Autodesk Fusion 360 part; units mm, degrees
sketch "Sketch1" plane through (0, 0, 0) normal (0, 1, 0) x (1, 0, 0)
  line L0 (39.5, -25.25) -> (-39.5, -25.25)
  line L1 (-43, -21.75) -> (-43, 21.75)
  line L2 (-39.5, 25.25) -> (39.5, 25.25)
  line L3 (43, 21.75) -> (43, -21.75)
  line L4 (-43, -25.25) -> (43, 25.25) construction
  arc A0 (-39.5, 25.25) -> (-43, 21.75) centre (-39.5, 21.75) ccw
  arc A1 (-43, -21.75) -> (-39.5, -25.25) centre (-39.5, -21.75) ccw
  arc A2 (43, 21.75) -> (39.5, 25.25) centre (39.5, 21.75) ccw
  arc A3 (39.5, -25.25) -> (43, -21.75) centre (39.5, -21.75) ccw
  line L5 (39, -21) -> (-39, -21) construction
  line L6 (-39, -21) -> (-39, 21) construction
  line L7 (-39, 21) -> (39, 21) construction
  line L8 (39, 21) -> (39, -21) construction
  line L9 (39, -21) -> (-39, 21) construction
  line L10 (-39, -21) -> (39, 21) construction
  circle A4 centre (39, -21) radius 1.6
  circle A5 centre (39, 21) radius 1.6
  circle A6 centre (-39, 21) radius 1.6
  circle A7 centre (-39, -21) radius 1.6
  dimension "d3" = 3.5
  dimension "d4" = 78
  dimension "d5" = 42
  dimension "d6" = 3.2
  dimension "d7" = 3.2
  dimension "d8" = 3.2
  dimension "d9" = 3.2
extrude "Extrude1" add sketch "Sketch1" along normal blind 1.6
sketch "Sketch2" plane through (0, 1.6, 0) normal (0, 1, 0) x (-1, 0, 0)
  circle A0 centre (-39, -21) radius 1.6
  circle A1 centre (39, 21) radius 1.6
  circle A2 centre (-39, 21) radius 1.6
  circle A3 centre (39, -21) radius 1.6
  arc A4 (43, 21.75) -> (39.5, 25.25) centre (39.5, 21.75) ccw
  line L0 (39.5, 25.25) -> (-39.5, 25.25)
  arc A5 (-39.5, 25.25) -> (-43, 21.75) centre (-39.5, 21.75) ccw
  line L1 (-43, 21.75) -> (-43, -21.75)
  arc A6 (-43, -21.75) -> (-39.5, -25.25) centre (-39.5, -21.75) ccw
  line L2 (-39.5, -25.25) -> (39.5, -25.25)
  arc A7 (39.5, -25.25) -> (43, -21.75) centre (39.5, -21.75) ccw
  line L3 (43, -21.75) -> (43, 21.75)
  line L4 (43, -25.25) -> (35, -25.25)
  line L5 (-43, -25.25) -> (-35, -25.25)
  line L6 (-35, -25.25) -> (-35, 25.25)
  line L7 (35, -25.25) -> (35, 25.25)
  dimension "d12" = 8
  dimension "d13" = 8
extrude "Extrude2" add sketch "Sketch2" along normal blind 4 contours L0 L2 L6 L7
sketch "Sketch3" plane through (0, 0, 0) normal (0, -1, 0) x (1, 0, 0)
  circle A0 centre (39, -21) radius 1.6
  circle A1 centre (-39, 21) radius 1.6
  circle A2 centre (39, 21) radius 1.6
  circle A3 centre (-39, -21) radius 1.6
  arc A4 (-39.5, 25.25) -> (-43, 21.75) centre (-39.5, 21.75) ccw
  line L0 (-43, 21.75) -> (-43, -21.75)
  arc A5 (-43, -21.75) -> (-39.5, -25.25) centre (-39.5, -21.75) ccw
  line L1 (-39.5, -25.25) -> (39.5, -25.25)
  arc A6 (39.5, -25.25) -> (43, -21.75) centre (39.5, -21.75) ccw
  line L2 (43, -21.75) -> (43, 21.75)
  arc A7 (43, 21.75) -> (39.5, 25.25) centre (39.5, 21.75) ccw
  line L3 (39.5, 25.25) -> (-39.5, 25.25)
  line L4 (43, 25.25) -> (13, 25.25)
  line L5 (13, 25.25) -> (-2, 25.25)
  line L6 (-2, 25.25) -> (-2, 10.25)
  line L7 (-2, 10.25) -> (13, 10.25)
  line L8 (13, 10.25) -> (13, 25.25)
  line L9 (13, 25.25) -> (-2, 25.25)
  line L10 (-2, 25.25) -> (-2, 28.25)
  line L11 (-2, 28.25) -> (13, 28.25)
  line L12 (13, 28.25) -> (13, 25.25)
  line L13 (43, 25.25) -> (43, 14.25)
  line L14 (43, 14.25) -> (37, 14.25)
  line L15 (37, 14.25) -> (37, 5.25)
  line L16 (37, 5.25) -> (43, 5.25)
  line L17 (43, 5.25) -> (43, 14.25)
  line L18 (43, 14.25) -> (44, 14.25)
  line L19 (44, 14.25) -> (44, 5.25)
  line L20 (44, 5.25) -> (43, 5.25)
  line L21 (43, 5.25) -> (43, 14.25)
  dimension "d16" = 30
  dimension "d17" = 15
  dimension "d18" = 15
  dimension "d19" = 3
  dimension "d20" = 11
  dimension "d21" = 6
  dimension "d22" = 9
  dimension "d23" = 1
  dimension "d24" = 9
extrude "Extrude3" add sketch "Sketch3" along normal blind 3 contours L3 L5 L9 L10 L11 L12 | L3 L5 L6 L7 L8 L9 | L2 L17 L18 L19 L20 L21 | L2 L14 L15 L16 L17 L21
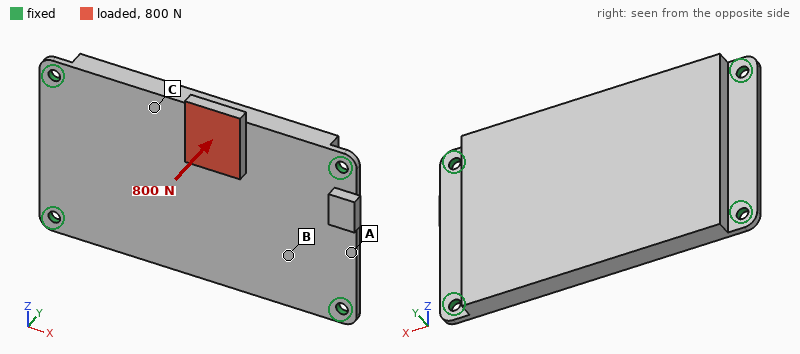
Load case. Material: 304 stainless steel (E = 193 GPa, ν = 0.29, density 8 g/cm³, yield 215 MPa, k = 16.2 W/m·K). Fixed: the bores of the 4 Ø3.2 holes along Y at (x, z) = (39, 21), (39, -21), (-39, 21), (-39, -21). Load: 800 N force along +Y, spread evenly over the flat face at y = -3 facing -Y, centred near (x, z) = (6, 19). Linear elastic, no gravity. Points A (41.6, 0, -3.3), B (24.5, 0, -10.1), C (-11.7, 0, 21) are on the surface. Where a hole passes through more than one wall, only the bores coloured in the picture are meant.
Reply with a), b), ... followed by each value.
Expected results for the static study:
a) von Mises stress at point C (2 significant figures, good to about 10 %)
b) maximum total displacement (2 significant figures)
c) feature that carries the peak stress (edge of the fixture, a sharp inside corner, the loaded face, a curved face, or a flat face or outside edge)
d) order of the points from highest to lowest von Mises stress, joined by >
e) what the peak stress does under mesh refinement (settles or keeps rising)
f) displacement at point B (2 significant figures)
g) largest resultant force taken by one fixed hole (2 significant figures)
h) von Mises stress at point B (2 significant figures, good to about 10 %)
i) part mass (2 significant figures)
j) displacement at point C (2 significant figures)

a) 33 MPa
b) 57 µm
c) edge of the fixture
d) C > B > A
e) keeps rising
f) 11 µm
g) 920 N
h) 17 MPa
i) 180 g
j) 40 µm
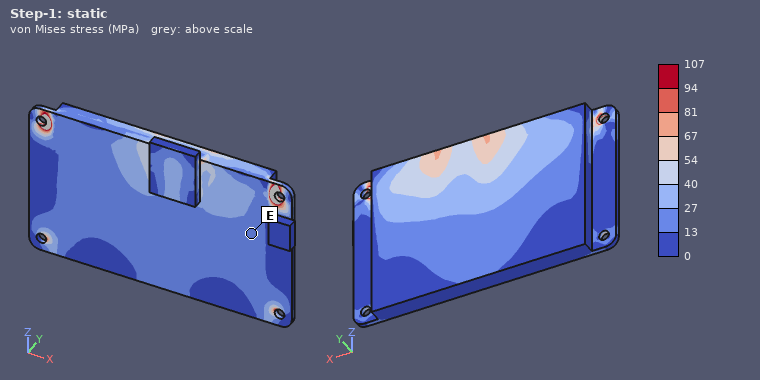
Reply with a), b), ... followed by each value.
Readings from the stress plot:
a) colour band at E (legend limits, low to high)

a) 13 to 27 MPa
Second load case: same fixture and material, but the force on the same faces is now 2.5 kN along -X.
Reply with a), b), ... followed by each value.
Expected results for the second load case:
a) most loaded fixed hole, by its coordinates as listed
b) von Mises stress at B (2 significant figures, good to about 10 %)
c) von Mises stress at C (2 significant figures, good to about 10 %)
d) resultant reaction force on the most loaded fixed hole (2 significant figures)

a) (39, 21)
b) 14 MPa
c) 43 MPa
d) 920 N
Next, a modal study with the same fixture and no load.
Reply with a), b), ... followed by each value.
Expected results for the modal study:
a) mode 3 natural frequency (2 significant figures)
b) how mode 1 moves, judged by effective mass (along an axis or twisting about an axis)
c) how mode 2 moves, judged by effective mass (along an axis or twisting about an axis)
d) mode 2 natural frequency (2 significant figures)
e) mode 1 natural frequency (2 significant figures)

a) 6600 Hz
b) along Y
c) twisting about X
d) 4500 Hz
e) 2700 Hz
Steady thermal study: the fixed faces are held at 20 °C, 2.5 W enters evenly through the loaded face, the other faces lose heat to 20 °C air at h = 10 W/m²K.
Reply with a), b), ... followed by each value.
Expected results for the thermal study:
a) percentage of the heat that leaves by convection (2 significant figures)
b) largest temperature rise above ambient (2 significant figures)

a) 37 %
b) 24 K
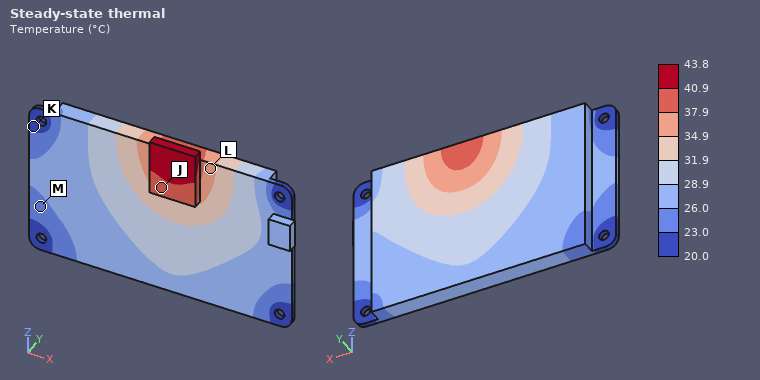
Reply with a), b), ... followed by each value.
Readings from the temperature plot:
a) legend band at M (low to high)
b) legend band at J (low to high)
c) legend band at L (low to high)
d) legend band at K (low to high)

a) 23.0 to 26.0 °C
b) 37.9 to 40.9 °C
c) 34.9 to 37.9 °C
d) 20.0 to 23.0 °C
